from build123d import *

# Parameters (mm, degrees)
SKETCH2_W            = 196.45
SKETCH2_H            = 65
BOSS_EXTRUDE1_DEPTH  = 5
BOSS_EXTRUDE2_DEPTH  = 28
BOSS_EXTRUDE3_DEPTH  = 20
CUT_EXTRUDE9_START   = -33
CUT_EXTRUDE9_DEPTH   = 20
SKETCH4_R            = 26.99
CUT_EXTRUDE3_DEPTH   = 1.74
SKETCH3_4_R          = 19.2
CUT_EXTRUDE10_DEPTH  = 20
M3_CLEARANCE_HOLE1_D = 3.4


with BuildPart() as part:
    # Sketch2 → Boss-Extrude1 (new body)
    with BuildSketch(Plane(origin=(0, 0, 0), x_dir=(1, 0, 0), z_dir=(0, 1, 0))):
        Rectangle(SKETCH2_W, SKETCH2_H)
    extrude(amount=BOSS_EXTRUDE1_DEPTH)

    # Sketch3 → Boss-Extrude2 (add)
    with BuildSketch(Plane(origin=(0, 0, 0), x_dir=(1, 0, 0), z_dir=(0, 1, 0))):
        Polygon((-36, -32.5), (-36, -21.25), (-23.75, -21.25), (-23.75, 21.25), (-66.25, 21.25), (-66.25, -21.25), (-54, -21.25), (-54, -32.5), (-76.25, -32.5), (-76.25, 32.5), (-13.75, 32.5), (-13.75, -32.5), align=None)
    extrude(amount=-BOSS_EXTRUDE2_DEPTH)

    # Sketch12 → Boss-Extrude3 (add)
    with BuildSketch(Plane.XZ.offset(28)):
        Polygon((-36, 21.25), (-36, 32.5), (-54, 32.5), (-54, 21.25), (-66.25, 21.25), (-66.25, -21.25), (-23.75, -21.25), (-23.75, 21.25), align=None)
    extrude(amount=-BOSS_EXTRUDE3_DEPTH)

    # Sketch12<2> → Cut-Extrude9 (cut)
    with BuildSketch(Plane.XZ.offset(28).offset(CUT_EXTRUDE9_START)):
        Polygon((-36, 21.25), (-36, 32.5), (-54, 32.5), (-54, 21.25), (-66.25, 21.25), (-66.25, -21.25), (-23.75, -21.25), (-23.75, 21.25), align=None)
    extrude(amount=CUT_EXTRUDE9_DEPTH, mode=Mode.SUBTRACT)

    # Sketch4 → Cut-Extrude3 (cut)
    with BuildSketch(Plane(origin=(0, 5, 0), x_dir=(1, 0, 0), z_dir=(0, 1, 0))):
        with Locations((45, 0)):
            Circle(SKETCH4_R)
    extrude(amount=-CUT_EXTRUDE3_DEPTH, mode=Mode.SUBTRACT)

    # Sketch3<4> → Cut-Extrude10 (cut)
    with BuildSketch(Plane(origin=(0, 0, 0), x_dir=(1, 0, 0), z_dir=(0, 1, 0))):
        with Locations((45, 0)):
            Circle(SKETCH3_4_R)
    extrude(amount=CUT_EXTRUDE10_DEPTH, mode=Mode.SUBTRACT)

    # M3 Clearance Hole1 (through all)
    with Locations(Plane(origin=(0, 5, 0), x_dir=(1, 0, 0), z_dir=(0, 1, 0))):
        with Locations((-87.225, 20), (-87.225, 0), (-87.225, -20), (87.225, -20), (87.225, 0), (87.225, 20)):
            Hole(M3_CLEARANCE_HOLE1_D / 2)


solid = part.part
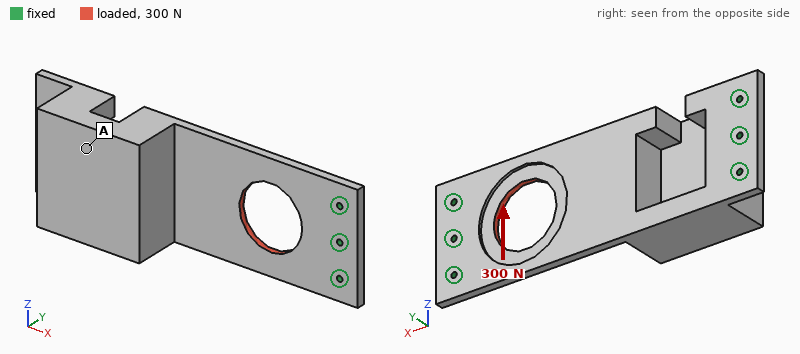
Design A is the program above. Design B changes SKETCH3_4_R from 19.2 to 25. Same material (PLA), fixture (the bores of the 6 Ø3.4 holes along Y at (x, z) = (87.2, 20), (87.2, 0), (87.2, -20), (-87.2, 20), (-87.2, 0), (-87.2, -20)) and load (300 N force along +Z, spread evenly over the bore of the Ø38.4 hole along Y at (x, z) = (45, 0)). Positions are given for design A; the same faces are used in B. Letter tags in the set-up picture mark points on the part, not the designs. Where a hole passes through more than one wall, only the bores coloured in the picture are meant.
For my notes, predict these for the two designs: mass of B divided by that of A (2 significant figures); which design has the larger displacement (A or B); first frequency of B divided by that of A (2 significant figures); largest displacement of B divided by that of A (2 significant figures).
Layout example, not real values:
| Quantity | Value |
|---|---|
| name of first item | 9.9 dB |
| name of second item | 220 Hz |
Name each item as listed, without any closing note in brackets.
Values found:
| Quantity | Value |
|---|---|
| mass of B divided by that of A | 0.98 |
| which design has the larger displacement | B |
| first frequency of B divided by that of A | 0.97 |
| largest displacement of B divided by that of A | 1.5 |
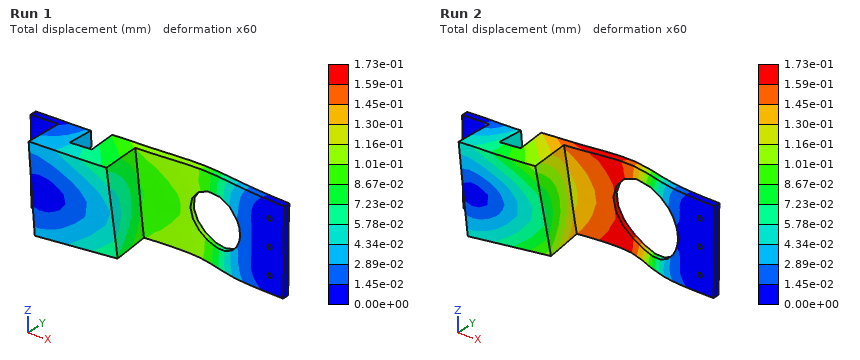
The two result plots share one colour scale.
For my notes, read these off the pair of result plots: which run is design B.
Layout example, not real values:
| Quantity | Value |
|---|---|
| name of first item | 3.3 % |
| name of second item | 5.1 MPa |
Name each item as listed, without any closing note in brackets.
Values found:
| Quantity | Value |
|---|---|
| which run is design B | Run 2 |
